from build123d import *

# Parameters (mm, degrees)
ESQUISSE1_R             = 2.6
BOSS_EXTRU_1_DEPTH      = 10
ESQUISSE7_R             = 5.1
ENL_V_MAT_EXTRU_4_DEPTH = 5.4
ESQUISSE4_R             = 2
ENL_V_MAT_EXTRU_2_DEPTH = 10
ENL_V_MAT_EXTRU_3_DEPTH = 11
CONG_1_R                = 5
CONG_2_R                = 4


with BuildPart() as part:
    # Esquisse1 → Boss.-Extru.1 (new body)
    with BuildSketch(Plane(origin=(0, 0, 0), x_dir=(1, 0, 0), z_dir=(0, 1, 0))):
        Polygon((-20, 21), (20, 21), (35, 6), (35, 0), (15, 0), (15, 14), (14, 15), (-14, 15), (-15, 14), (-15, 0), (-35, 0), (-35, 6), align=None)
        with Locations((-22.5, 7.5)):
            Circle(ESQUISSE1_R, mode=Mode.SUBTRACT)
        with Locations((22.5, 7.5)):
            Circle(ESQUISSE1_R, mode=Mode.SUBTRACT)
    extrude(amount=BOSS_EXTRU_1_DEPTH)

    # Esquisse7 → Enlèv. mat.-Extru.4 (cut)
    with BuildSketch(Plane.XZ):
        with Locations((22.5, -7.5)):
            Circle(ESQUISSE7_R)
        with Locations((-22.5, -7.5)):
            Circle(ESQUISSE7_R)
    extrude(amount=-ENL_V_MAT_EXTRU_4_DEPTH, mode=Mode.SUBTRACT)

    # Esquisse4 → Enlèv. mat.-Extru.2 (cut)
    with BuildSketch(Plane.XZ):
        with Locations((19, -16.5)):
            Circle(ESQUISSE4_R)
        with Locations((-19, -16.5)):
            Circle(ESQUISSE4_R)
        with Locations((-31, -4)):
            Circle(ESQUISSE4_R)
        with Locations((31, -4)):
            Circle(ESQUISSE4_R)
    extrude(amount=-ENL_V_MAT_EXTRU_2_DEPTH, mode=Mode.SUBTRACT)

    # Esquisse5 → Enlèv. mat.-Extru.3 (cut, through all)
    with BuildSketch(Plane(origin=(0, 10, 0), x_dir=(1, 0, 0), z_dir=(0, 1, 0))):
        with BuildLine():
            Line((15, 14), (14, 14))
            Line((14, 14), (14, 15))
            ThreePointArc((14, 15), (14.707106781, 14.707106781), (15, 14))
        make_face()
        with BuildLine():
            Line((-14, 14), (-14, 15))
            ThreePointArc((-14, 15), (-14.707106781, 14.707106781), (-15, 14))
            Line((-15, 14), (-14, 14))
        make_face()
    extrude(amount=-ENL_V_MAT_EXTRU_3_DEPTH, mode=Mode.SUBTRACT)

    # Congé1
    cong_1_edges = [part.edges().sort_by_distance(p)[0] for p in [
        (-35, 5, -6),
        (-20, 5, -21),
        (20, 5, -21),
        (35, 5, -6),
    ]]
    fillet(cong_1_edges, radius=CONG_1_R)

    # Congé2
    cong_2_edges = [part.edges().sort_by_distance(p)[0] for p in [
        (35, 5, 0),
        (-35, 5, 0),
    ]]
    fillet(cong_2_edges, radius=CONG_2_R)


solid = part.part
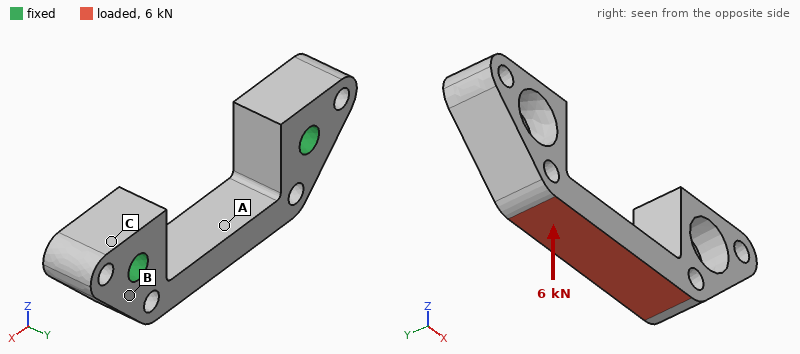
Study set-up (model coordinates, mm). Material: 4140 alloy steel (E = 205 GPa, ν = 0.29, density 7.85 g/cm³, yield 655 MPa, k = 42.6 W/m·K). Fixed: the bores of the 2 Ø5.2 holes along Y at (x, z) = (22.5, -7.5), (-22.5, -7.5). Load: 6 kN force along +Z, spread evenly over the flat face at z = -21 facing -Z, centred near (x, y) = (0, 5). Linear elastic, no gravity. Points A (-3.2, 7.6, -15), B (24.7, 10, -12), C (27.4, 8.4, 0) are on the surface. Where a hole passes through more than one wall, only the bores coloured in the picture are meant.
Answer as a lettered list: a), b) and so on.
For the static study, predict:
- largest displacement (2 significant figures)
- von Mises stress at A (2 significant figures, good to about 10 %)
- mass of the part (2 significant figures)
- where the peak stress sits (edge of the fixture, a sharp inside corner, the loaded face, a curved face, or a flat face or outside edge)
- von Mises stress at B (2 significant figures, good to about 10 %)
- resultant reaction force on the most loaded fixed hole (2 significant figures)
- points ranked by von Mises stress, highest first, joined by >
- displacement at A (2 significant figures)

a) 42 µm
b) 110 MPa
c) 49 g
d) a curved face
e) 63 MPa
f) 3.7 kN
g) A > B > C
h) 33 µm
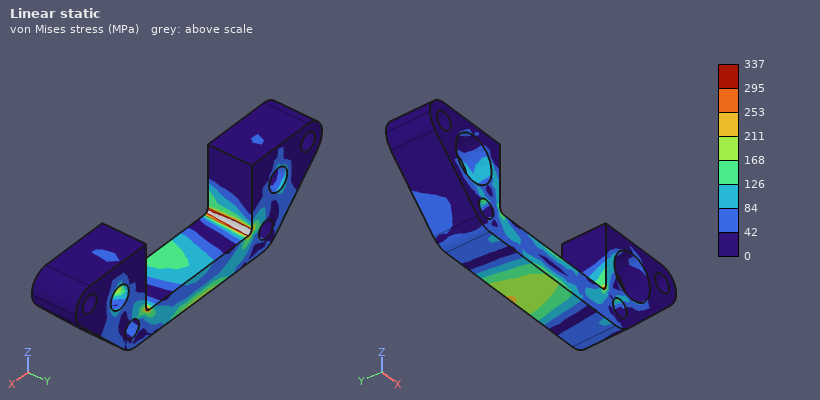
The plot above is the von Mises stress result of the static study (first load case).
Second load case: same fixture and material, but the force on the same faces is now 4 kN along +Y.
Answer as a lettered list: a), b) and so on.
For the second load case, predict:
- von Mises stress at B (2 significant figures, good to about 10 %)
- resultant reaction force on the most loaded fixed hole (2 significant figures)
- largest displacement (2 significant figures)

a) 170 MPa
b) 2.0 kN
c) 67 µm
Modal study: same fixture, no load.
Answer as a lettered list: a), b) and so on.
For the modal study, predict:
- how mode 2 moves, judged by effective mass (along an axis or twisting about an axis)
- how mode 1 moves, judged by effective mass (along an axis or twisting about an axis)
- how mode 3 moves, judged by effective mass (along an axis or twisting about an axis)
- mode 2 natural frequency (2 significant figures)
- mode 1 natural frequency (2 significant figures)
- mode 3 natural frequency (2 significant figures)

a) along Z
b) along Y
c) along X
d) 19 kHz
e) 12 kHz
f) 20 kHz
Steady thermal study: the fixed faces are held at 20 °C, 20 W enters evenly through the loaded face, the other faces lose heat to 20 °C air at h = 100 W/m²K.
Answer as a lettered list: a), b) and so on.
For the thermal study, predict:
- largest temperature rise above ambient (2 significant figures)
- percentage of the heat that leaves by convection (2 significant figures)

a) 57 K
b) 28 %
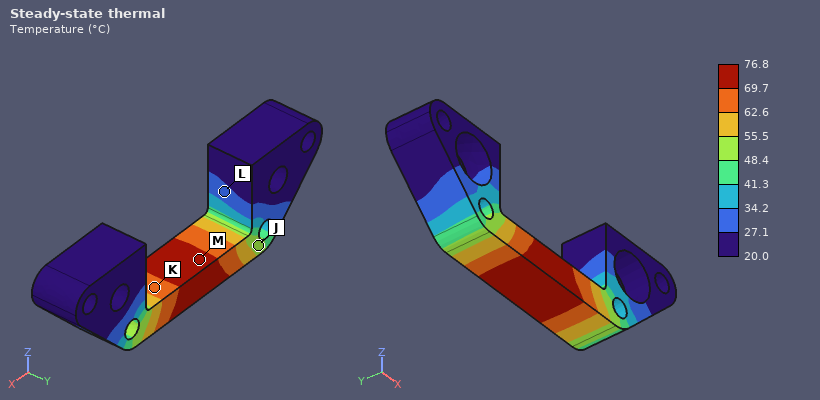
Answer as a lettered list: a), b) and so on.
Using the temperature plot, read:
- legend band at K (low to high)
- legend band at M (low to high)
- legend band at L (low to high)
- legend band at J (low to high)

a) 62.6 to 69.7 °C
b) 69.7 to 76.8 °C
c) 27.1 to 34.2 °C
d) 48.4 to 55.5 °C
